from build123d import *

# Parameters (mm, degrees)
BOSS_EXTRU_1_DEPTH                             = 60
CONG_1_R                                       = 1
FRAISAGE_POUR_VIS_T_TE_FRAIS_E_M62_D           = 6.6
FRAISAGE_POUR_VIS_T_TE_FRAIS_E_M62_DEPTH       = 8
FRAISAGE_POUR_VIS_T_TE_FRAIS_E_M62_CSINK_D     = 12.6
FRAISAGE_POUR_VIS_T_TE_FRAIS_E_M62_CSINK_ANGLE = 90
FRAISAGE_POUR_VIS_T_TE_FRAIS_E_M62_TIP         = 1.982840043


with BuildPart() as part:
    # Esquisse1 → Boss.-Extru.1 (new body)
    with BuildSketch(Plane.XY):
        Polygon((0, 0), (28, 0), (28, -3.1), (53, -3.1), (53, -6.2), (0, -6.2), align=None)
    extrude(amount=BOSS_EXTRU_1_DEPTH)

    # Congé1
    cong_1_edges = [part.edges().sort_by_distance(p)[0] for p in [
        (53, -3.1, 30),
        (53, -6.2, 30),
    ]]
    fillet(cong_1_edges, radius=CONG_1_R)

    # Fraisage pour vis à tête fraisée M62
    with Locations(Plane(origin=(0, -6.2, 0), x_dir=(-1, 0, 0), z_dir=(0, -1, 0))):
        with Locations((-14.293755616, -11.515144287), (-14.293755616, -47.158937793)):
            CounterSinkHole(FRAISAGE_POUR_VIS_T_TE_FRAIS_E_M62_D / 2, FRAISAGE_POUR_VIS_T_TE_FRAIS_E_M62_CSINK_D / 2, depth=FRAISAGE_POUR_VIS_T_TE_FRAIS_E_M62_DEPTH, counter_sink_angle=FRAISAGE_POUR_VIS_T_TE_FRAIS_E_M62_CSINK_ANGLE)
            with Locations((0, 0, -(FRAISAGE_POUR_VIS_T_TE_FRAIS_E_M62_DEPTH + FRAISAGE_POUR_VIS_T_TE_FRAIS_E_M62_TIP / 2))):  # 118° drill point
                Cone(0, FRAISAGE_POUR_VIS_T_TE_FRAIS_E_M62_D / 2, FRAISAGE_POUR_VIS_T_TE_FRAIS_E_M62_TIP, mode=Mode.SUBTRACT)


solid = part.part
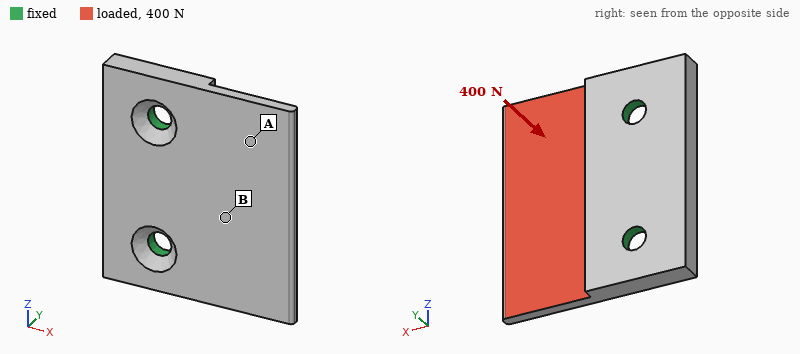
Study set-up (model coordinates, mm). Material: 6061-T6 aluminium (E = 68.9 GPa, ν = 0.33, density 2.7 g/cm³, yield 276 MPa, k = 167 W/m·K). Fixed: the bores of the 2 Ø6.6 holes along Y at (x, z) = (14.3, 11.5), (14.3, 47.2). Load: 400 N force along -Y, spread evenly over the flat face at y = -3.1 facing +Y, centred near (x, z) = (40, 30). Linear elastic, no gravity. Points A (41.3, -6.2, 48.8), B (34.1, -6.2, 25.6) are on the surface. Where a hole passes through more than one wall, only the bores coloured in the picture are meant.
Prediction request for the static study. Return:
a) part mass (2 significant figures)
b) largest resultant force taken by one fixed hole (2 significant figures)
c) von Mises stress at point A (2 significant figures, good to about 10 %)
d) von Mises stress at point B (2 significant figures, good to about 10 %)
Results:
39 g
220 N
9.1 MPa
25 MPa
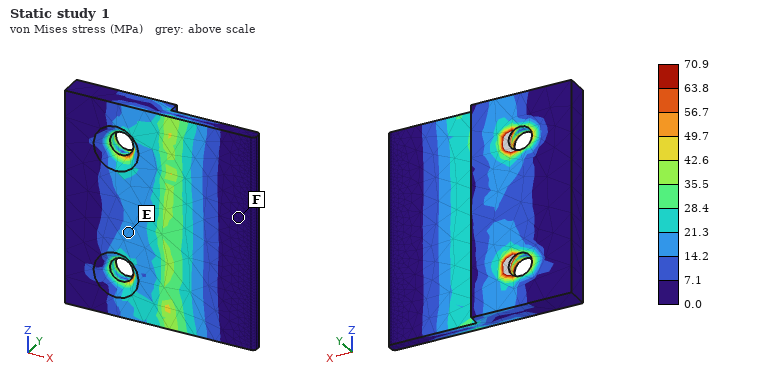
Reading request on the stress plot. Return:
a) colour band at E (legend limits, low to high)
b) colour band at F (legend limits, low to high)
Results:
14.2 to 21.3 MPa
0.0 to 7.1 MPa
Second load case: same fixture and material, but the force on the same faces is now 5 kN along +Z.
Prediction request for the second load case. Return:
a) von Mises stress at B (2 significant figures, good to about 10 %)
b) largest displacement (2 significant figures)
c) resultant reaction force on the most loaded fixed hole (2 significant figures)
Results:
33 MPa
0.15 mm
4.1 kN
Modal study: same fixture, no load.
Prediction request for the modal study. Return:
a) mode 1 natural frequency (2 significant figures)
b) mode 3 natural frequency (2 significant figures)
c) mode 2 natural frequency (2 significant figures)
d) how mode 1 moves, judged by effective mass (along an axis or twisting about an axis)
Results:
2800 Hz
8000 Hz
4300 Hz
along Y
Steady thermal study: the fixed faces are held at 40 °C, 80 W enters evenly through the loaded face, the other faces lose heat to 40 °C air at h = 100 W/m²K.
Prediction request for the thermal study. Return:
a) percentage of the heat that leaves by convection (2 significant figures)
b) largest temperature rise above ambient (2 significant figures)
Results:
14 %
49 K
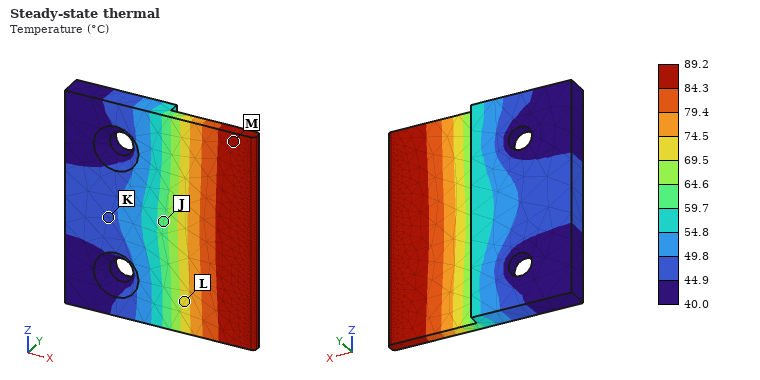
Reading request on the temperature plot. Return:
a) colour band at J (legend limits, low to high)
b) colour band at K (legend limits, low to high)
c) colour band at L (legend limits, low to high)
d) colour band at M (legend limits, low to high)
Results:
59.7 to 64.6 °C
44.9 to 49.8 °C
69.5 to 74.5 °C
84.3 to 89.2 °C
